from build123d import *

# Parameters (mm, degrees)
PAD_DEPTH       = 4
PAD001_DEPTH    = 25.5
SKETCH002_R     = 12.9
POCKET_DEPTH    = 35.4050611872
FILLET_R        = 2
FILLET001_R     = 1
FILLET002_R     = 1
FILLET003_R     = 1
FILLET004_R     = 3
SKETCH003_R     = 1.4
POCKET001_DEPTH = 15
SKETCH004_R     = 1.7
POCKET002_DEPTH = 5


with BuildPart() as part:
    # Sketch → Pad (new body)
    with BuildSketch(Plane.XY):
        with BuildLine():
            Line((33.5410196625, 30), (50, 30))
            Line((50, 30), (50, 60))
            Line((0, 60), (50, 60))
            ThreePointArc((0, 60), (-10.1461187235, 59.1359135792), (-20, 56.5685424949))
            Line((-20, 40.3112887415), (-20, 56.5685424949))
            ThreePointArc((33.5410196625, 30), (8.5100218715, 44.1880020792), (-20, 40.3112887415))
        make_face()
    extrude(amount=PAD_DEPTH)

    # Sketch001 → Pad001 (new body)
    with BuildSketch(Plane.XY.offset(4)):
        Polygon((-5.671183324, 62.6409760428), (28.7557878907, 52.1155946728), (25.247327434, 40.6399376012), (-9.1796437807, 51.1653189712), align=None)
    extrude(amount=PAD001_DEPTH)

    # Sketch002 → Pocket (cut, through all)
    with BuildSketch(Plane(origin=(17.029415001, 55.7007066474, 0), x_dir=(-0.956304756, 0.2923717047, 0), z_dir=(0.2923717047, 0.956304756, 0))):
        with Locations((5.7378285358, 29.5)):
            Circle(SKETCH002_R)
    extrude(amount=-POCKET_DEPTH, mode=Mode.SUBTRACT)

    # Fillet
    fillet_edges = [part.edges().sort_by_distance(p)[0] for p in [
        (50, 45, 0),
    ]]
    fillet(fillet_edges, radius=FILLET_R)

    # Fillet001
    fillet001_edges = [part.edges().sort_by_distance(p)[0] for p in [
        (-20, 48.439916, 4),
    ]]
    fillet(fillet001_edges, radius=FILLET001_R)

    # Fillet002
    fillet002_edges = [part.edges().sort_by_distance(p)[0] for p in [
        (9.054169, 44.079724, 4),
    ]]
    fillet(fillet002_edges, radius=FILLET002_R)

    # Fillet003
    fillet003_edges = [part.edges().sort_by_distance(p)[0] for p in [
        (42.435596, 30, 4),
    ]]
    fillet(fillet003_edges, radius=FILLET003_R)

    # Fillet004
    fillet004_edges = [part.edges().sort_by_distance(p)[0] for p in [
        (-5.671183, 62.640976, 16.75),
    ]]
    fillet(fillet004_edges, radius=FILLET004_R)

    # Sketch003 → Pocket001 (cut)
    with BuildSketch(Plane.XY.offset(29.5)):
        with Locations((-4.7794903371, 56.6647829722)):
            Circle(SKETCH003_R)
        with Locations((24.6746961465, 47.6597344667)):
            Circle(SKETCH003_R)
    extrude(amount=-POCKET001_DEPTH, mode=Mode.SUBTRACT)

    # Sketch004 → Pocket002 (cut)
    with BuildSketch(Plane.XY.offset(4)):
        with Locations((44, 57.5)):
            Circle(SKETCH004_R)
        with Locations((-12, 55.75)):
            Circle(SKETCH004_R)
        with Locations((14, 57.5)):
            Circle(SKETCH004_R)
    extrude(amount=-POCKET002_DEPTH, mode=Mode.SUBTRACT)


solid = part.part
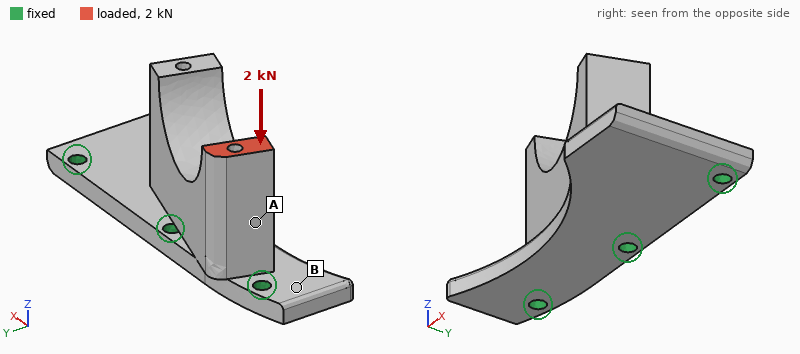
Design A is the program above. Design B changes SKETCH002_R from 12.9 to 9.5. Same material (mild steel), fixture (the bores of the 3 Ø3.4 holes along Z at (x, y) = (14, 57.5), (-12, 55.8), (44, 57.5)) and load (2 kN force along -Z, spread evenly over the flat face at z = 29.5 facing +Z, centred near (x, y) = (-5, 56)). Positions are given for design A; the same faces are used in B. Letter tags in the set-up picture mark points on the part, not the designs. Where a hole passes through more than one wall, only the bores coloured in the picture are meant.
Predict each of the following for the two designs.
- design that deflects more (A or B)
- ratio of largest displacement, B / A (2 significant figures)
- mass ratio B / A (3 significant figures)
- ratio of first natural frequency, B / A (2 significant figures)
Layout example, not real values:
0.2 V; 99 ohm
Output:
A; 0.67; 1.11; 0.88
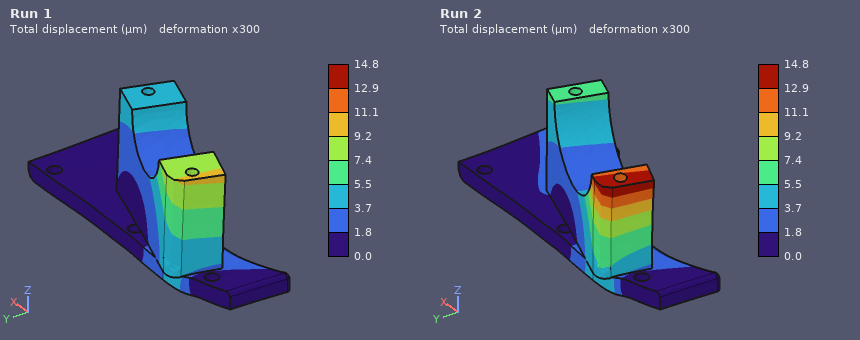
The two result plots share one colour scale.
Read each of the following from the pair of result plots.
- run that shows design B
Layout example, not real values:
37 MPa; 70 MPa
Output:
Run 1
